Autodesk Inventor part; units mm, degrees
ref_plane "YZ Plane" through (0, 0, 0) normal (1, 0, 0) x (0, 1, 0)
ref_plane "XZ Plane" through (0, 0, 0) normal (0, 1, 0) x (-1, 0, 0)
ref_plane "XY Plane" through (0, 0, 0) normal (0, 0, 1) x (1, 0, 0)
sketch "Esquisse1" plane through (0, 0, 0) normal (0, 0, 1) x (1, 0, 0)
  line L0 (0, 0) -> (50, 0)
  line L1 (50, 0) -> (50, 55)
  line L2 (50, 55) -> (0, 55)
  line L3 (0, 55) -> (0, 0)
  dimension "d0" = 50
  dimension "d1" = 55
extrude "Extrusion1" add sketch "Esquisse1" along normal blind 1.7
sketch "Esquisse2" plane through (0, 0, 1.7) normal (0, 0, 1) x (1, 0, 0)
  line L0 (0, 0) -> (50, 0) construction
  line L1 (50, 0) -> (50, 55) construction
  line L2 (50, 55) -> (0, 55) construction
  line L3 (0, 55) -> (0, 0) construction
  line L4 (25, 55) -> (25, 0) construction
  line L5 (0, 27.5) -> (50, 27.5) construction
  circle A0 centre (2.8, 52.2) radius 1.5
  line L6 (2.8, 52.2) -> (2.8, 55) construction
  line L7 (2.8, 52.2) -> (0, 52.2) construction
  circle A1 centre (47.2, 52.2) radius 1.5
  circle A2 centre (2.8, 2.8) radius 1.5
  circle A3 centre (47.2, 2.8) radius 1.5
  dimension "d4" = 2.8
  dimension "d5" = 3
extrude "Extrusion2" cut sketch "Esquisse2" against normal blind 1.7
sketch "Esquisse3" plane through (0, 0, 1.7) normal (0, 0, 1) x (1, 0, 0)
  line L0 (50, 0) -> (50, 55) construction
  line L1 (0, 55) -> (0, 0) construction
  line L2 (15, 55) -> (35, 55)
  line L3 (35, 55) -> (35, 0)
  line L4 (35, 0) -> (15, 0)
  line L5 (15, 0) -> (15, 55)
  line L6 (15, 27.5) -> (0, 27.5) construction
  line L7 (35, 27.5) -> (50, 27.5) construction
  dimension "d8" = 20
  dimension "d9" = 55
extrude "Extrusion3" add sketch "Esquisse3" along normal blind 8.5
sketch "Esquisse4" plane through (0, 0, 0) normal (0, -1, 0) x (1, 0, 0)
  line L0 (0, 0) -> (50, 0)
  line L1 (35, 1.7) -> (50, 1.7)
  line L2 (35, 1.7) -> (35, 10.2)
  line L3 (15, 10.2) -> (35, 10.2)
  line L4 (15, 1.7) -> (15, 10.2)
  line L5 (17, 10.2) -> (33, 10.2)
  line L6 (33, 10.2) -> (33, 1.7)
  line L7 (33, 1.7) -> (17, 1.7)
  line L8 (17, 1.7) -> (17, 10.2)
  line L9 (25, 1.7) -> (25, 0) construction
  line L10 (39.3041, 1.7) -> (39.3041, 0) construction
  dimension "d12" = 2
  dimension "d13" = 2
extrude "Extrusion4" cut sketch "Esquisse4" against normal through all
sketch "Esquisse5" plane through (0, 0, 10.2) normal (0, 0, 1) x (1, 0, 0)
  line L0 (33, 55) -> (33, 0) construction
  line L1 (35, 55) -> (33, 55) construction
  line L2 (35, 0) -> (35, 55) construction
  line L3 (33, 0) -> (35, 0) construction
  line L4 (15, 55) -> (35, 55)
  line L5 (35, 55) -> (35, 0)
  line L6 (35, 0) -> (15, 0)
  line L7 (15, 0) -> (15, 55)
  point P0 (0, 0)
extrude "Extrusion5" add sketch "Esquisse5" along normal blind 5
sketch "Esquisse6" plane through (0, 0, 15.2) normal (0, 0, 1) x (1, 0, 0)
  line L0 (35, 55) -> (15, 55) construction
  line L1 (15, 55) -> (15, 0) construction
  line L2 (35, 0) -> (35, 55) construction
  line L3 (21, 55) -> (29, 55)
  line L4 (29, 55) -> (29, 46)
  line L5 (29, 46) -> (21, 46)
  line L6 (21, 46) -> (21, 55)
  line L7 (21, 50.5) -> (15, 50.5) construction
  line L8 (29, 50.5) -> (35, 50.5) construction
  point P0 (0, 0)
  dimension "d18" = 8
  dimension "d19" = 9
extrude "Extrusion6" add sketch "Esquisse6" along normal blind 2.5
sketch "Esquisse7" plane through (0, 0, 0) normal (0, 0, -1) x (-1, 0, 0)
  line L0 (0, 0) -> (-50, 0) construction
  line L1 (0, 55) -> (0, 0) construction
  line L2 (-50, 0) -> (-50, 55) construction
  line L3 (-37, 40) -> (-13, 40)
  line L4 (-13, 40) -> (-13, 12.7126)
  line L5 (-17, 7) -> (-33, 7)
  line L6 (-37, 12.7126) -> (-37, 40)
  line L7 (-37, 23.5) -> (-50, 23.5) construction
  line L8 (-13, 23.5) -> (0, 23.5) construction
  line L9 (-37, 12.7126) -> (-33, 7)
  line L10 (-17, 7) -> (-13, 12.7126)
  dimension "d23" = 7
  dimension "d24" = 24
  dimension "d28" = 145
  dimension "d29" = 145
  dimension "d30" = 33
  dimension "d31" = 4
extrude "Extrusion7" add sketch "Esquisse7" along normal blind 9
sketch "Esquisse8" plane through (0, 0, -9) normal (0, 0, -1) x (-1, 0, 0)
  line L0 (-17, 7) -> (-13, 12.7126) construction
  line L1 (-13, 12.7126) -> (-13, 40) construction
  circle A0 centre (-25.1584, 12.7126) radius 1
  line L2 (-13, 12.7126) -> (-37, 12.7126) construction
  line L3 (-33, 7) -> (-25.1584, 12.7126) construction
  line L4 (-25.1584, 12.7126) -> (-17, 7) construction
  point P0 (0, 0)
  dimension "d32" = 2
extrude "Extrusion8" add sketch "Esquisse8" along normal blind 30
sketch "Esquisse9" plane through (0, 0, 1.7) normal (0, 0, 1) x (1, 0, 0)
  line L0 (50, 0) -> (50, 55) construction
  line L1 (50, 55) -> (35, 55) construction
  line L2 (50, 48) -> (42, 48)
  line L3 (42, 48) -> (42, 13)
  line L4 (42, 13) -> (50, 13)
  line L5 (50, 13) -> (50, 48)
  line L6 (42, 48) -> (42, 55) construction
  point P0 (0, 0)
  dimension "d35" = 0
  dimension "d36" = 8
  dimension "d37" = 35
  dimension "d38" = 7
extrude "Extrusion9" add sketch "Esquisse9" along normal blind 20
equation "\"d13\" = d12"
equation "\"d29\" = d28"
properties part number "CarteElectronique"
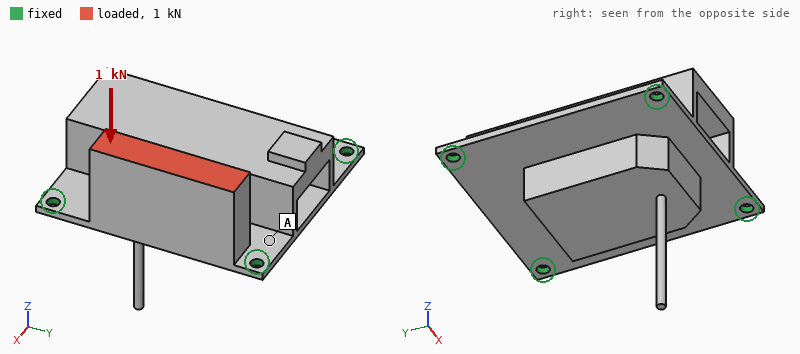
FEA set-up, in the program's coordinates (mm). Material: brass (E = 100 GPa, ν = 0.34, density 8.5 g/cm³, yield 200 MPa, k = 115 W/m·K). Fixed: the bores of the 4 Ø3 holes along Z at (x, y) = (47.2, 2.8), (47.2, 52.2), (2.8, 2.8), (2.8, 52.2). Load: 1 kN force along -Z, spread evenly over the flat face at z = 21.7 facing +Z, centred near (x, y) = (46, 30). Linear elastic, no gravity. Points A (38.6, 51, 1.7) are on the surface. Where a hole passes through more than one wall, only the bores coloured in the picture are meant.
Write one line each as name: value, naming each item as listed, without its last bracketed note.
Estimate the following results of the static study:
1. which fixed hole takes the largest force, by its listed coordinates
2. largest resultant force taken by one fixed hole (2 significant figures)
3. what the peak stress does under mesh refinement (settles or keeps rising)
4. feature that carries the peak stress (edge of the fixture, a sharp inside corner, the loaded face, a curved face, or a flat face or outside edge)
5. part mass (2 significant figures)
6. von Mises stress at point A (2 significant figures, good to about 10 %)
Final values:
which fixed hole takes the largest force, by its listed coordinates: (47.2, 52.2)
largest resultant force taken by one fixed hole: 650 N
what the peak stress does under mesh refinement: keeps rising
feature that carries the peak stress: edge of the fixture
part mass: 210 g
von Mises stress at point A: 25 MPa
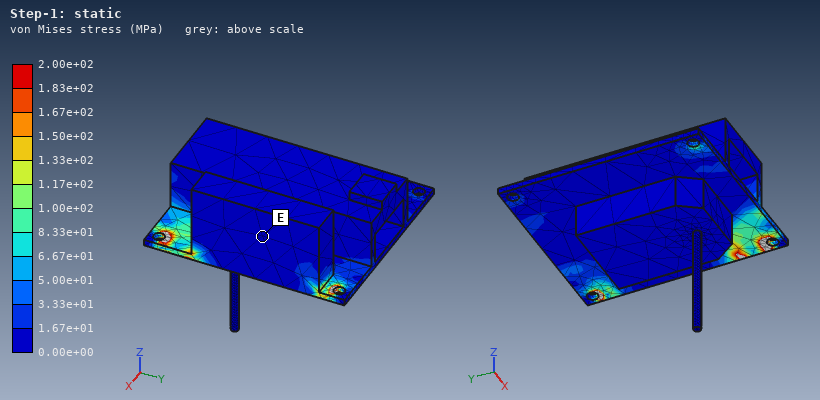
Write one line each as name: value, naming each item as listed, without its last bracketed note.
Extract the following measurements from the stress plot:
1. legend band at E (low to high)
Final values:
legend band at E: 0.00e+00 to 1.67e+01 MPa
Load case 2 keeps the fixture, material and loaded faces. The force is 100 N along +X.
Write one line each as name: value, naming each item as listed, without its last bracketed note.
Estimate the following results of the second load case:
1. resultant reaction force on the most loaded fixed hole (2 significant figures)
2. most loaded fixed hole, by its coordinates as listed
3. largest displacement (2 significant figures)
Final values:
resultant reaction force on the most loaded fixed hole: 58 N
most loaded fixed hole, by its coordinates as listed: (47.2, 52.2)
largest displacement: 64 µm
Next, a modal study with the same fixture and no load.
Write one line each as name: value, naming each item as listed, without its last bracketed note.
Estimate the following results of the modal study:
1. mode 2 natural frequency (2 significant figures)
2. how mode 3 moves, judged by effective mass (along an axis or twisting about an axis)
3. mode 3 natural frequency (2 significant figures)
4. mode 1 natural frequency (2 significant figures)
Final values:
mode 2 natural frequency: 1000 Hz
how mode 3 moves, judged by effective mass: along Z
mode 3 natural frequency: 1300 Hz
mode 1 natural frequency: 1000 Hz
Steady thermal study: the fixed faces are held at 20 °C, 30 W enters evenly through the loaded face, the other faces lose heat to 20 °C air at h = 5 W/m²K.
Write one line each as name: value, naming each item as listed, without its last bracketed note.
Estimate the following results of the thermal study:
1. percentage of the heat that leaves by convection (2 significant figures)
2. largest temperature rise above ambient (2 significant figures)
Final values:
percentage of the heat that leaves by convection: 5.6 %
largest temperature rise above ambient: 60 K
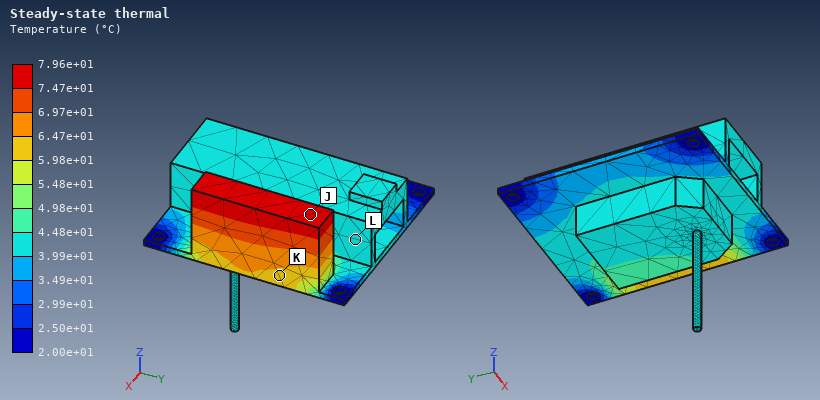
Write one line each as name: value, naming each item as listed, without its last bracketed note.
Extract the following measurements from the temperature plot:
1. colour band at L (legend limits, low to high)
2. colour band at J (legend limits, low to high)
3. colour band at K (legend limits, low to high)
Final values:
colour band at L: 3.99e+01 to 4.48e+01 °C
colour band at J: 7.47e+01 to 7.96e+01 °C
colour band at K: 5.98e+01 to 6.47e+01 °C
